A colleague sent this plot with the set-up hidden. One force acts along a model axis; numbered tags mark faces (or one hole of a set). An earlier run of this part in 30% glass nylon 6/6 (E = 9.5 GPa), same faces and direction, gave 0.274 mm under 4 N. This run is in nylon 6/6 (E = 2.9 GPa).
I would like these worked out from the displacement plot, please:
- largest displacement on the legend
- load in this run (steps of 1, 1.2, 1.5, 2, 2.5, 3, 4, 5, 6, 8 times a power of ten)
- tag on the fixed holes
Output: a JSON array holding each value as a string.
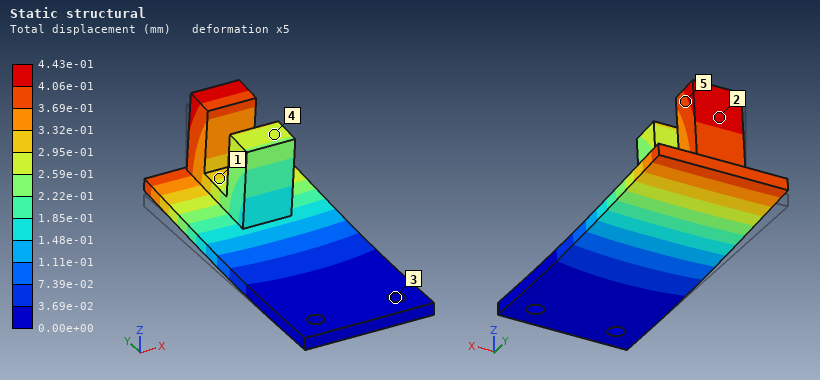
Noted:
["4.43e-01 mm", "2 N", "3"]
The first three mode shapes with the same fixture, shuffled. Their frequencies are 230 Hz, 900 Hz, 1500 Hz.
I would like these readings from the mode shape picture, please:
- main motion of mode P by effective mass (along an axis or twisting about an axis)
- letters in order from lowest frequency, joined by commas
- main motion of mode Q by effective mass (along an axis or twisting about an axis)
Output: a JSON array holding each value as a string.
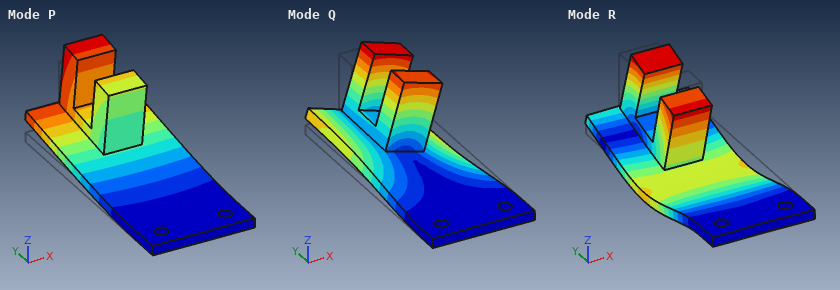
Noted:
["along Z", "P, Q, R", "along X"]
